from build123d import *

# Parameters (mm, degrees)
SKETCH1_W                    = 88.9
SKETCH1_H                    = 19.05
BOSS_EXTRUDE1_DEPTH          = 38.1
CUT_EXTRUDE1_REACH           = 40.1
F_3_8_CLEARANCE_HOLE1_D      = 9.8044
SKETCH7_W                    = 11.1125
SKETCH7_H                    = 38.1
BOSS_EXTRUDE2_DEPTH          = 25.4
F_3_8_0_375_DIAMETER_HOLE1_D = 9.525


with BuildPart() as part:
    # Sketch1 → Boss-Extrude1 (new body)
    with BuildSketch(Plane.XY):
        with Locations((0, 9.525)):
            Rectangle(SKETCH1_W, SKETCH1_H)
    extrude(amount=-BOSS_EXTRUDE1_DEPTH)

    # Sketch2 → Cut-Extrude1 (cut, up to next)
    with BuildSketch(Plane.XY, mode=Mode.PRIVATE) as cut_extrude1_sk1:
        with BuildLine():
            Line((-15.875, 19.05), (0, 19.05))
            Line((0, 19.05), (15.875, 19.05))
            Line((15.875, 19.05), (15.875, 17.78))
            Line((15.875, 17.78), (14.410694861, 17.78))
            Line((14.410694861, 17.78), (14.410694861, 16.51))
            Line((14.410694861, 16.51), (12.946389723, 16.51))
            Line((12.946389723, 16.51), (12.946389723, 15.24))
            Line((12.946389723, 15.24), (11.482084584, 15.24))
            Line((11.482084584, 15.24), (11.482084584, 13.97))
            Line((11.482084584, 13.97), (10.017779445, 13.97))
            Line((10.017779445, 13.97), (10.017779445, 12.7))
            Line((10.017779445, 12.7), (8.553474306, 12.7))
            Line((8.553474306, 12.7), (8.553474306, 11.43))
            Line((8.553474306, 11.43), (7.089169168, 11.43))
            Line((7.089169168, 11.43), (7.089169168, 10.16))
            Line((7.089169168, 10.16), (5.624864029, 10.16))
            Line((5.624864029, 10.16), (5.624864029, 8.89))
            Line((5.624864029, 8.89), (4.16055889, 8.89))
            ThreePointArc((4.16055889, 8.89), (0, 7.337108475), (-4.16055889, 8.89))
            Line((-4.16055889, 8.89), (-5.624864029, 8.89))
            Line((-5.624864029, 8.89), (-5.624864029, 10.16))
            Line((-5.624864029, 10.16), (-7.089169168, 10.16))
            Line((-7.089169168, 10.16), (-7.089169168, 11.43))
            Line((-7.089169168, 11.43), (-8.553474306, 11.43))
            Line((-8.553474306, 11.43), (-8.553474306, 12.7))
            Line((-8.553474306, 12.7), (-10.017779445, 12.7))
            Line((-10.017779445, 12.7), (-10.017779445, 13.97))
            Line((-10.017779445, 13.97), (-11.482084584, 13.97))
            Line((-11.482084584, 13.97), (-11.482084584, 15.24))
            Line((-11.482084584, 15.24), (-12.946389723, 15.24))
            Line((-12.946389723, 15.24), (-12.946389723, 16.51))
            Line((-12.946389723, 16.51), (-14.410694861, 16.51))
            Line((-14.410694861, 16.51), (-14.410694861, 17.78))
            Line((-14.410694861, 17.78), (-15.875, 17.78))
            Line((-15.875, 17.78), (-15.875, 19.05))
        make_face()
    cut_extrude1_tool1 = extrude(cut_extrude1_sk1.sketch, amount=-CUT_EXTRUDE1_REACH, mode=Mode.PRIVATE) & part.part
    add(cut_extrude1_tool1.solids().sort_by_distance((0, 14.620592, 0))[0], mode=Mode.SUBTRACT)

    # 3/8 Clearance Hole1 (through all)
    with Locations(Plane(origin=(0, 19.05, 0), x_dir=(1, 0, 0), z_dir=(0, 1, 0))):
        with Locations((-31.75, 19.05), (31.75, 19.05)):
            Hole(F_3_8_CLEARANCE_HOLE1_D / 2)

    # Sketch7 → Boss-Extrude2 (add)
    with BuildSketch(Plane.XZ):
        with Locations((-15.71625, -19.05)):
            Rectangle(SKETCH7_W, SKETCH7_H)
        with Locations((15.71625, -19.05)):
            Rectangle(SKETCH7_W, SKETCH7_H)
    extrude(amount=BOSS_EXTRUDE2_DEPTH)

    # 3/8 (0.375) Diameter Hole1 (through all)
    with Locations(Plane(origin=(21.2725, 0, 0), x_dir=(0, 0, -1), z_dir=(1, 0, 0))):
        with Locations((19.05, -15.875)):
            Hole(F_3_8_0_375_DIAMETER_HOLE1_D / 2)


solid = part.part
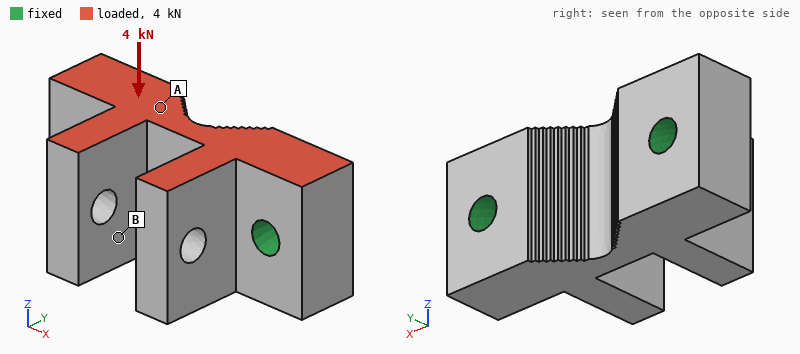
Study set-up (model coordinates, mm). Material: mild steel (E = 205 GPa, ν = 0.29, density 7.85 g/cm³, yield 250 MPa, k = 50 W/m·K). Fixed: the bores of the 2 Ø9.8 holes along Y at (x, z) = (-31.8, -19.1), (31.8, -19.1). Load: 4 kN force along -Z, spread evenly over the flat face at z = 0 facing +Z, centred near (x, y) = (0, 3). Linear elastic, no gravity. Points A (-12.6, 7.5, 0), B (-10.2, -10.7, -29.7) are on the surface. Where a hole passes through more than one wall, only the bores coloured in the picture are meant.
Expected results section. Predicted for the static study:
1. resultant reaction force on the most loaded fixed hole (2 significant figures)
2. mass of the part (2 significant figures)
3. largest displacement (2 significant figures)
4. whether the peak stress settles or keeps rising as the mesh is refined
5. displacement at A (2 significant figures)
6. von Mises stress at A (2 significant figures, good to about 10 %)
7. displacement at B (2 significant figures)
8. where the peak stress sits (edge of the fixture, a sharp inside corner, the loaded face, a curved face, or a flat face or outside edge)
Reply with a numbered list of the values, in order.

1. 2.0 kN
2. 570 g
3. 3.1 µm
4. keeps rising
5. 1.2 µm
6. 4.4 MPa
7. 1.7 µm
8. edge of the fixture
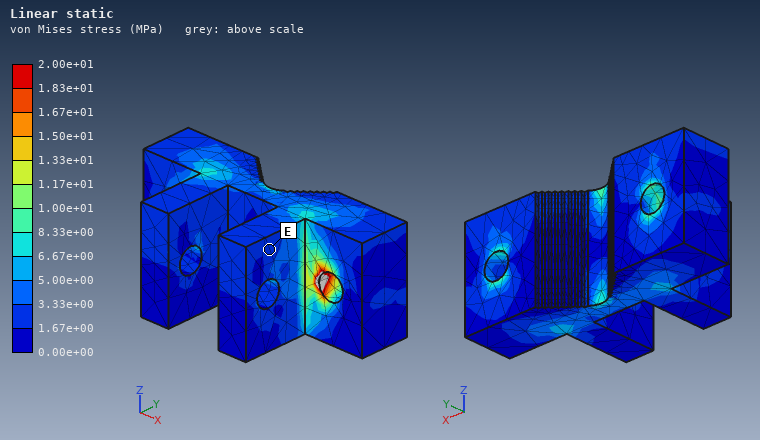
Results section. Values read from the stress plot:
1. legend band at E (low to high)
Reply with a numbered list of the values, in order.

1. 1.67e+00 to 3.33e+00 MPa
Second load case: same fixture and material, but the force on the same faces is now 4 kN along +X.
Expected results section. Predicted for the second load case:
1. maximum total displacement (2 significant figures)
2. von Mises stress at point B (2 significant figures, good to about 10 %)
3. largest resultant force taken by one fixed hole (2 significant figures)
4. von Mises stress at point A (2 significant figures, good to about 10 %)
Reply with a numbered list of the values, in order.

1. 6.1 µm
2. 4.4 MPa
3. 2.2 kN
4. 5.9 MPa
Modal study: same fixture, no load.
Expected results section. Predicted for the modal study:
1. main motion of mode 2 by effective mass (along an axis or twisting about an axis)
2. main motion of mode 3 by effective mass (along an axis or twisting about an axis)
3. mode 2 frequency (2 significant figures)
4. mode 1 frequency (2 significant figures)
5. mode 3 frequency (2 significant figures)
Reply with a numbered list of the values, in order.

1. along Z
2. along X
3. 9300 Hz
4. 8500 Hz
5. 9800 Hz
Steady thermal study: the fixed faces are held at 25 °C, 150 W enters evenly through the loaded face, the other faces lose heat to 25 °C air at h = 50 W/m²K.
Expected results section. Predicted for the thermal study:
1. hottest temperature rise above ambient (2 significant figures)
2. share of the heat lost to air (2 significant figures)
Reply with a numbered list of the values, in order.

1. 54 K
2. 9.9 %
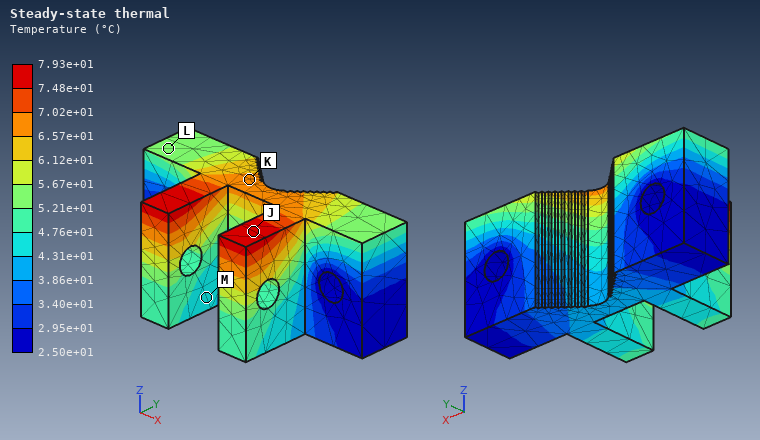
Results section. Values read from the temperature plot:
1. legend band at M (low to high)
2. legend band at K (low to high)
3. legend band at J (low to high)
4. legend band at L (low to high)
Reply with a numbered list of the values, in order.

1. 4.31e+01 to 4.76e+01 °C
2. 6.57e+01 to 7.02e+01 °C
3. 7.48e+01 to 7.93e+01 °C
4. 5.21e+01 to 5.67e+01 °C
